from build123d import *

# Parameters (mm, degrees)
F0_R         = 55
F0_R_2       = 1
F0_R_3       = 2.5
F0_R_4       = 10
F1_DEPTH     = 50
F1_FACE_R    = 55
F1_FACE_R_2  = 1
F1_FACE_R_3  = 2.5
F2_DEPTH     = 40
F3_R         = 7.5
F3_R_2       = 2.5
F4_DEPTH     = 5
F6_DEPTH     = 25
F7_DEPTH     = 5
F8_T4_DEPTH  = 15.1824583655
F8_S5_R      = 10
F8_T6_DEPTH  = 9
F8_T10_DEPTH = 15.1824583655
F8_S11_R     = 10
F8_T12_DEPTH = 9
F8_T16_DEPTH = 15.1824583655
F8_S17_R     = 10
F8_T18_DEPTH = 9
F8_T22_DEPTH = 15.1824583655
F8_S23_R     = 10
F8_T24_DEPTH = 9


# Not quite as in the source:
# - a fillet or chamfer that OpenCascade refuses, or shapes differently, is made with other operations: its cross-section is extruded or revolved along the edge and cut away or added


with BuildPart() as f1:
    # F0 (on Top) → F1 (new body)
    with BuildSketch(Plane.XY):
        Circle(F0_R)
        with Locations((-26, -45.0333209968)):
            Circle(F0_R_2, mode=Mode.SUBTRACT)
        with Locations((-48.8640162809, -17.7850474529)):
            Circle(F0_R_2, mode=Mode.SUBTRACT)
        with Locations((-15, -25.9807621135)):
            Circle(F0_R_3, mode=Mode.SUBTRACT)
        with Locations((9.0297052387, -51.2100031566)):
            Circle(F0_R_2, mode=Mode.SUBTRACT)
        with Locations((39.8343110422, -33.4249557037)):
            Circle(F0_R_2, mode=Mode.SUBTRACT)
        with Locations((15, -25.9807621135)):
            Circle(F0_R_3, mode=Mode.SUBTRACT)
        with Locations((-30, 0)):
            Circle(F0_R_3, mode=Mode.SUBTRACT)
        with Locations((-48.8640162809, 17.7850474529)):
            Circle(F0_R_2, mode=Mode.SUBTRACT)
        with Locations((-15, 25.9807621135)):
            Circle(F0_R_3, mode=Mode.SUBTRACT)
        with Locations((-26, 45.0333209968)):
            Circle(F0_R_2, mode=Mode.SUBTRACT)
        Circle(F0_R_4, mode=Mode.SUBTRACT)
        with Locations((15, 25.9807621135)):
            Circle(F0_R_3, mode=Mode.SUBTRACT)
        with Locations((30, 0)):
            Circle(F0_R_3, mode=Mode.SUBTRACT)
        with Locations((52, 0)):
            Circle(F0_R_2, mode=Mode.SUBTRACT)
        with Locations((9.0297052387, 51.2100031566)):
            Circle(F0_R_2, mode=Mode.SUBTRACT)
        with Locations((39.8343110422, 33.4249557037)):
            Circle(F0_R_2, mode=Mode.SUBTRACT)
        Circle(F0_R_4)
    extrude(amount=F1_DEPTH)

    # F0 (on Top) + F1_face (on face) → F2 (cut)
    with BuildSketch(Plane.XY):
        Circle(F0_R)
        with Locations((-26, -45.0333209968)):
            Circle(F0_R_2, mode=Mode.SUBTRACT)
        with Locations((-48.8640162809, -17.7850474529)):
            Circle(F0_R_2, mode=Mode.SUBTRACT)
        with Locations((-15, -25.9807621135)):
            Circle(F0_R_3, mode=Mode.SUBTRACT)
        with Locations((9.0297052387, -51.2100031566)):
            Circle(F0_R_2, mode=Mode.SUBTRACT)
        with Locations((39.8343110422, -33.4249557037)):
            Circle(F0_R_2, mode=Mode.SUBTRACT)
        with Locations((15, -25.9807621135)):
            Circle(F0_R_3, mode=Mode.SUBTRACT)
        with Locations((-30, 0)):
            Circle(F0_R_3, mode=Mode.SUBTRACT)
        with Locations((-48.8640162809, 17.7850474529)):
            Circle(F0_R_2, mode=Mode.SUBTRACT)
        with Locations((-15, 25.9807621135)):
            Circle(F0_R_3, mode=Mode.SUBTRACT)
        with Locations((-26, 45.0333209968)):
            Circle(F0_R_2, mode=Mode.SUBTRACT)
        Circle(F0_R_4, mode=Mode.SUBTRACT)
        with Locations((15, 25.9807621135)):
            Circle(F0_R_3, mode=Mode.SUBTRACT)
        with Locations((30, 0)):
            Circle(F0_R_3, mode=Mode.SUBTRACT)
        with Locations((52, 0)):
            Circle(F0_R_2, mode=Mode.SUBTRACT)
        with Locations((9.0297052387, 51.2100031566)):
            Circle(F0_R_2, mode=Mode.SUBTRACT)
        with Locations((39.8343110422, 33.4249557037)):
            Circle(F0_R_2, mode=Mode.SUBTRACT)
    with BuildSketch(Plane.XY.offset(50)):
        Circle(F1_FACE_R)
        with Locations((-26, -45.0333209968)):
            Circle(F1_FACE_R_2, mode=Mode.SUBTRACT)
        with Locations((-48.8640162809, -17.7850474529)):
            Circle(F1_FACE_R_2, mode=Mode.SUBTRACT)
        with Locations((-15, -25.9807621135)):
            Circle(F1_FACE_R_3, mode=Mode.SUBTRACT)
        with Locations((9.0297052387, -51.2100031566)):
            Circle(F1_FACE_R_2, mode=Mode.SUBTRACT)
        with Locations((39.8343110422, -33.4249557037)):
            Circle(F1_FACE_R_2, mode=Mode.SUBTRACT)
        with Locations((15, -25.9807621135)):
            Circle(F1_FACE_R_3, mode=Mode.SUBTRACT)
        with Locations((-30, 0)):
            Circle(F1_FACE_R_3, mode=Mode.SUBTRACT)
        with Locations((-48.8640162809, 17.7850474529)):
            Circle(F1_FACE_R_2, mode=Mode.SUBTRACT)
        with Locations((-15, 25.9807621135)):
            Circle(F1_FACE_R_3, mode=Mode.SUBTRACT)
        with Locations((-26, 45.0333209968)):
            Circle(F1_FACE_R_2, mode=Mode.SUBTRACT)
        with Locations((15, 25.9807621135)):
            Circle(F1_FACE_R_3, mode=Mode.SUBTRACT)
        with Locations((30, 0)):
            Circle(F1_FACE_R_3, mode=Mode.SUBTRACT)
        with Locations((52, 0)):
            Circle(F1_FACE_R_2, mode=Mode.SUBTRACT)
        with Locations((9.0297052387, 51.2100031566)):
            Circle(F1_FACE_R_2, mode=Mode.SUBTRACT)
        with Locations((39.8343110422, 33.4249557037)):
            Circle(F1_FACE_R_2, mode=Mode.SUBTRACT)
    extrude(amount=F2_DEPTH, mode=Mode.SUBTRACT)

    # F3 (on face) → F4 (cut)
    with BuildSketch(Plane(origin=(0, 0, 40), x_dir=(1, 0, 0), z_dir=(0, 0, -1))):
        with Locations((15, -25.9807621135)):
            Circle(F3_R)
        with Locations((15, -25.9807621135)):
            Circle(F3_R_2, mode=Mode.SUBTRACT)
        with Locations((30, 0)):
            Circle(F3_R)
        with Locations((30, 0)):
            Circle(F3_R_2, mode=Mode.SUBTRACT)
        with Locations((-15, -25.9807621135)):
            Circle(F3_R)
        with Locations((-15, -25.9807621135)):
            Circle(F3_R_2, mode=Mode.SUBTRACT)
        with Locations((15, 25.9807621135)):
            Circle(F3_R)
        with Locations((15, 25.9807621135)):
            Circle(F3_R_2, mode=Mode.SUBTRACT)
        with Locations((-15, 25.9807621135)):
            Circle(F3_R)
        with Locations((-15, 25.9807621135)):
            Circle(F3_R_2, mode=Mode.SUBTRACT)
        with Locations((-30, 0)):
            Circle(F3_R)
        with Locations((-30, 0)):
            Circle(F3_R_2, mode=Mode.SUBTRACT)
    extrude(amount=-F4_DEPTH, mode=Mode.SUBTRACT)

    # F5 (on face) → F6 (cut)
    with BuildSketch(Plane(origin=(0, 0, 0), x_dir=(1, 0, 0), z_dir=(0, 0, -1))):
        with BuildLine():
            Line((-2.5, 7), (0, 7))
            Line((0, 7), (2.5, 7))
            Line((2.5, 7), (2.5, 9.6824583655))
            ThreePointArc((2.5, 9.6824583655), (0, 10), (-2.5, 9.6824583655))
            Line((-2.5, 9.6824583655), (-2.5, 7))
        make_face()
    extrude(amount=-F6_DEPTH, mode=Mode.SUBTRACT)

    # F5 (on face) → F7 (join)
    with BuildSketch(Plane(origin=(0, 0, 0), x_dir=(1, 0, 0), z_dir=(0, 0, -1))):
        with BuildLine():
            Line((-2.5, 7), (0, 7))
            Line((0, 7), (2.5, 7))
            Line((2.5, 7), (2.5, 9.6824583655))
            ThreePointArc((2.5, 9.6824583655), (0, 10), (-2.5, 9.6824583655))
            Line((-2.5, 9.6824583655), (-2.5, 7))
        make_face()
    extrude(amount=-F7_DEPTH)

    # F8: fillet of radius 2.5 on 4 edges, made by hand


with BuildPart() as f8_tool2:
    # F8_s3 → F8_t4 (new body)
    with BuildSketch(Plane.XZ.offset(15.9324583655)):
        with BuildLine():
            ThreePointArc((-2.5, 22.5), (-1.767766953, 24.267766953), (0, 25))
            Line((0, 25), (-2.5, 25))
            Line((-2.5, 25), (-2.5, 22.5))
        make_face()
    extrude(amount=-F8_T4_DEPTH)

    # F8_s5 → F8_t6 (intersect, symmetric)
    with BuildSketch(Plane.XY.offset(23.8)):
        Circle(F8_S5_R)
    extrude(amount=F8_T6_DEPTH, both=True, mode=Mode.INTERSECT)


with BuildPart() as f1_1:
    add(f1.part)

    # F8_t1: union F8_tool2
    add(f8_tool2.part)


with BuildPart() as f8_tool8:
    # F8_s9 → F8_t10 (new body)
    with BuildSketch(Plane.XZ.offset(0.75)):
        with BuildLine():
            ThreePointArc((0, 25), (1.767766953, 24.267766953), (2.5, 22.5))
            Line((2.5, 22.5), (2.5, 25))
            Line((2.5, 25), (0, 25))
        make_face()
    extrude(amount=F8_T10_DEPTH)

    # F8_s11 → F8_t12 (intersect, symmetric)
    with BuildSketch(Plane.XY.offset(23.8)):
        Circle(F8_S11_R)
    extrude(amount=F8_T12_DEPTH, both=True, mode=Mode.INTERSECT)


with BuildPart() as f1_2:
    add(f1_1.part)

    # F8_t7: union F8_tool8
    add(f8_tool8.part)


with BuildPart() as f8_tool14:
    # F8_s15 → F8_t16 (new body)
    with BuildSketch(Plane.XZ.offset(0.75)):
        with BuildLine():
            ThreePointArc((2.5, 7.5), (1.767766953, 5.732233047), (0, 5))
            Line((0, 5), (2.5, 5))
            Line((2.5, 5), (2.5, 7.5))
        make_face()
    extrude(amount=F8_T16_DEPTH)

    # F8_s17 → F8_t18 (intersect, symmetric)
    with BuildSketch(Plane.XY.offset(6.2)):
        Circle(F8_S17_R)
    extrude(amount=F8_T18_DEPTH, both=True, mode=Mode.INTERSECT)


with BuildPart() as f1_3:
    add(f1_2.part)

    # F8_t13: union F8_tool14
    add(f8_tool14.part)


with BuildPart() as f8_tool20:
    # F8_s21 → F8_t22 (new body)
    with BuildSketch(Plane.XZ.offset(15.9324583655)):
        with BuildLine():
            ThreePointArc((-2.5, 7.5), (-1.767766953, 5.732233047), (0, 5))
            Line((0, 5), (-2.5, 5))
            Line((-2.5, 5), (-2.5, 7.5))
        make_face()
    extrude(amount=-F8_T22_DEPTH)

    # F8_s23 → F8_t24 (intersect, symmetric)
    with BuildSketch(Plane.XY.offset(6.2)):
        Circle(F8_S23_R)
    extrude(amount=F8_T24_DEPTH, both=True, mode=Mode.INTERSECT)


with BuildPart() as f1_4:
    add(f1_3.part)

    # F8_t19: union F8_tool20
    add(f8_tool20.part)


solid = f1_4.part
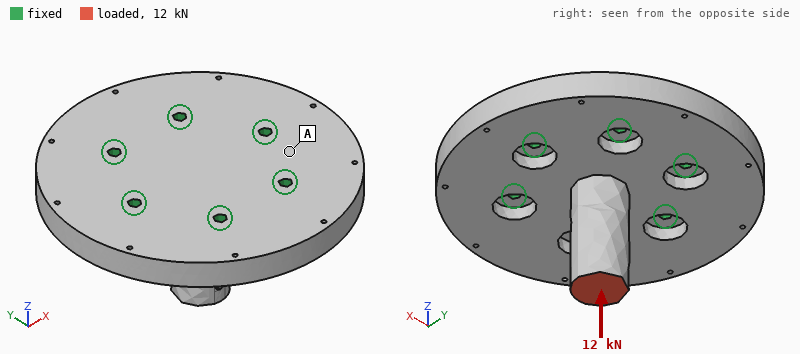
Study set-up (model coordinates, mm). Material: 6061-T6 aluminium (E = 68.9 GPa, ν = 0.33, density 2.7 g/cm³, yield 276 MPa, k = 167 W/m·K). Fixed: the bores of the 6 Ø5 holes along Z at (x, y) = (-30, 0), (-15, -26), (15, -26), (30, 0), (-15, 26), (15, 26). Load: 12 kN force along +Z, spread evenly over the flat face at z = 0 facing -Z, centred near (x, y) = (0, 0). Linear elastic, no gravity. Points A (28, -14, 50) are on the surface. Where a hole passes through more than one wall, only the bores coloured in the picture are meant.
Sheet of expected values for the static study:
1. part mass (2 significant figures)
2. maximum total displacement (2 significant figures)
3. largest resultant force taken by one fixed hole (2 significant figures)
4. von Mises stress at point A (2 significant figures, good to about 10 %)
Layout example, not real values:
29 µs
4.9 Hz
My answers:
270 g
67 µm
2.9 kN
20 MPa
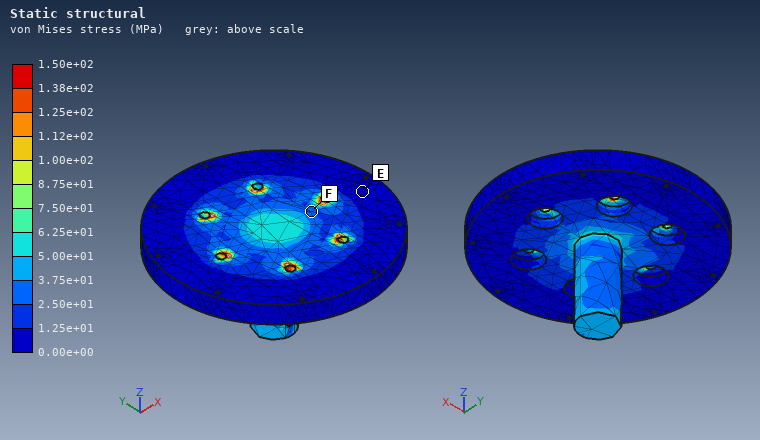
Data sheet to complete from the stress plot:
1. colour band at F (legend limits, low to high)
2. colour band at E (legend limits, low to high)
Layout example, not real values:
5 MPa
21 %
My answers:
2.50e+01 to 3.75e+01 MPa
0.00e+00 to 1.25e+01 MPa
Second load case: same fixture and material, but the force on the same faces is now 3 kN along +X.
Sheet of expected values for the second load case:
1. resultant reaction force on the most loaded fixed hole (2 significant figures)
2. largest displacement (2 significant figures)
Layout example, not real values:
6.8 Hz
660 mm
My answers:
2.1 kN
0.23 mm
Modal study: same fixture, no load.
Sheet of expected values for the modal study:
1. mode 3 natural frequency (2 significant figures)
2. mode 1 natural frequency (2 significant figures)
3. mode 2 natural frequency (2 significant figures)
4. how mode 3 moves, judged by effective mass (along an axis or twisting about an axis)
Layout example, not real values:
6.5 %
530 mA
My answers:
6800 Hz
5700 Hz
5800 Hz
along Z
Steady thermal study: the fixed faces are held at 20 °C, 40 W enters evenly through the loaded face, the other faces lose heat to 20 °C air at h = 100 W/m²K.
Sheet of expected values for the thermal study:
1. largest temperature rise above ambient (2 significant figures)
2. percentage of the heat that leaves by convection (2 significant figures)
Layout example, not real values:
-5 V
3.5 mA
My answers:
36 K
21 %
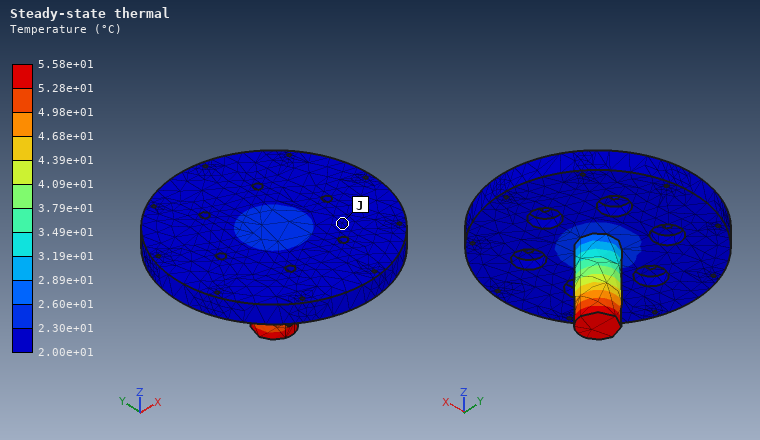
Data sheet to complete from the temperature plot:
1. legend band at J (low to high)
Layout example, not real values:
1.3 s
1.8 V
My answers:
2.00e+01 to 2.30e+01 °C
